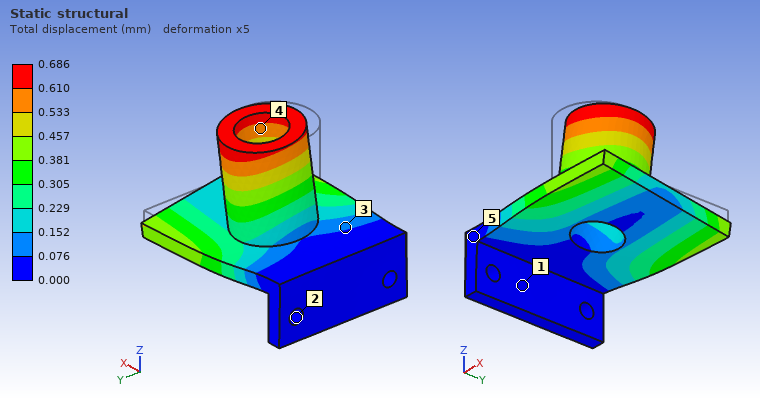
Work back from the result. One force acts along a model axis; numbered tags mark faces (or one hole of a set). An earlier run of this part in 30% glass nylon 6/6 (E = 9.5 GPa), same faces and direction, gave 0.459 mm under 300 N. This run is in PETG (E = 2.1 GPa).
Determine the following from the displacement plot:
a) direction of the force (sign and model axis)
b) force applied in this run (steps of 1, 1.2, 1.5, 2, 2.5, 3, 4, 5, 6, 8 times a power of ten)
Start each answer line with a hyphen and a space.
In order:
- +Y
- 100 N
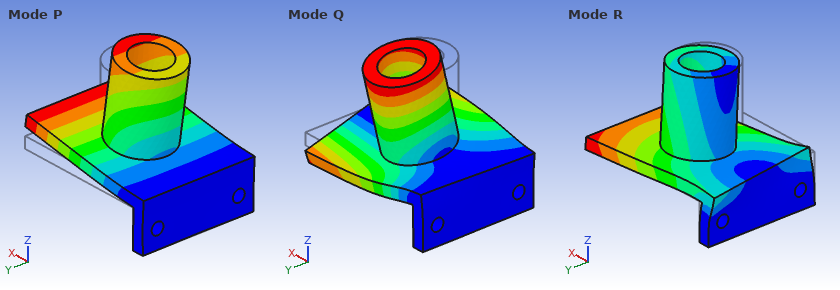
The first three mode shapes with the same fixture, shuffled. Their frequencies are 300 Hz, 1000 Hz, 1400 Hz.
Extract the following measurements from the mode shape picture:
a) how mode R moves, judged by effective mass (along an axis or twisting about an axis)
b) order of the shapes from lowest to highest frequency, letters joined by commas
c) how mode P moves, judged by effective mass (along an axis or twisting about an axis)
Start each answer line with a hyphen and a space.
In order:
- along Y
- P, Q, R
- along Z
